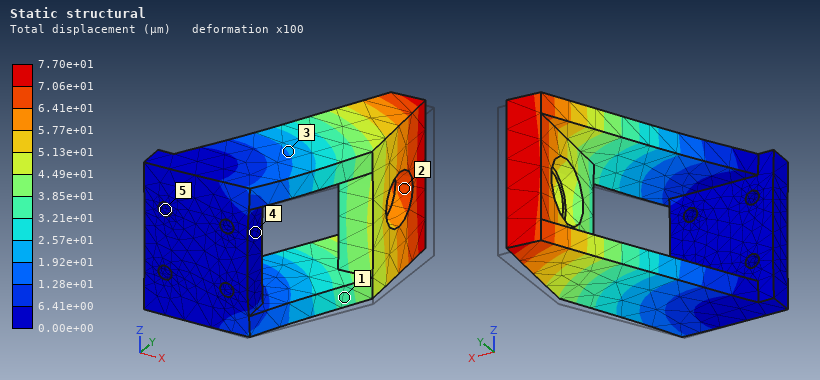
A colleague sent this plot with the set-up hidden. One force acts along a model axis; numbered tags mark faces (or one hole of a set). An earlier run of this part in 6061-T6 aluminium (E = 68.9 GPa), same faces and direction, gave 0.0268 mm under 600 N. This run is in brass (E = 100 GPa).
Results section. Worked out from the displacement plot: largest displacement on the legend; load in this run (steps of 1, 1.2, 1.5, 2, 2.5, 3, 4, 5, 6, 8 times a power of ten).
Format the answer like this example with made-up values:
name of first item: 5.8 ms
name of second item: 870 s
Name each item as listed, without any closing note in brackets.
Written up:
largest displacement on the legend: 7.70e+01 µm
load in this run: 2.5 kN
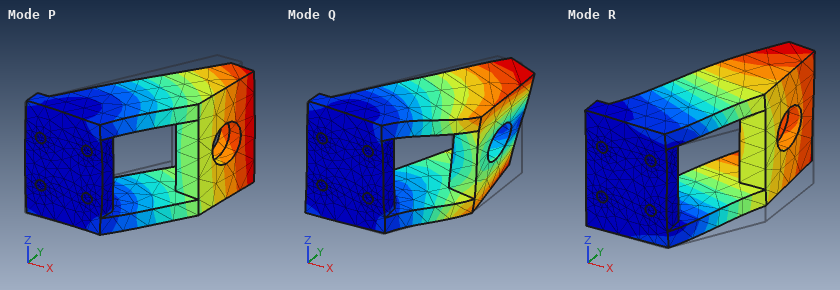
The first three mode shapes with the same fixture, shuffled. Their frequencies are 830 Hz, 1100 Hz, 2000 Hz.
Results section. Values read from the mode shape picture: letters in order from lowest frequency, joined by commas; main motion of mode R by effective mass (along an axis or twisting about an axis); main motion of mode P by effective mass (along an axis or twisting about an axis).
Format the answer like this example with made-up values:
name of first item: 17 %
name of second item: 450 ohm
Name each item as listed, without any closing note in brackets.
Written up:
letters in order from lowest frequency, joined by commas: R, P, Q
main motion of mode R by effective mass: along Z
main motion of mode P by effective mass: along X
